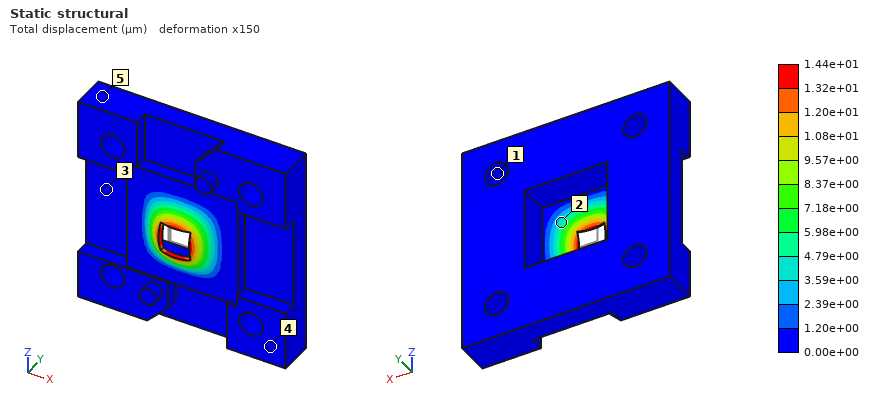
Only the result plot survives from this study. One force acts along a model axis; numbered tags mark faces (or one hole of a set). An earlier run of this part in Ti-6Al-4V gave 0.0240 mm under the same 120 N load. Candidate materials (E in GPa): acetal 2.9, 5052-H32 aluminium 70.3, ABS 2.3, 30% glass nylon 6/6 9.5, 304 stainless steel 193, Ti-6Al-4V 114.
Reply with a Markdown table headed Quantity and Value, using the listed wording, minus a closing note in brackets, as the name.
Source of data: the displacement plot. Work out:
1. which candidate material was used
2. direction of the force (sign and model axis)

| Quantity | Value |
|---|---|
| which candidate material was used | 304 stainless steel |
| direction of the force | -Y |
